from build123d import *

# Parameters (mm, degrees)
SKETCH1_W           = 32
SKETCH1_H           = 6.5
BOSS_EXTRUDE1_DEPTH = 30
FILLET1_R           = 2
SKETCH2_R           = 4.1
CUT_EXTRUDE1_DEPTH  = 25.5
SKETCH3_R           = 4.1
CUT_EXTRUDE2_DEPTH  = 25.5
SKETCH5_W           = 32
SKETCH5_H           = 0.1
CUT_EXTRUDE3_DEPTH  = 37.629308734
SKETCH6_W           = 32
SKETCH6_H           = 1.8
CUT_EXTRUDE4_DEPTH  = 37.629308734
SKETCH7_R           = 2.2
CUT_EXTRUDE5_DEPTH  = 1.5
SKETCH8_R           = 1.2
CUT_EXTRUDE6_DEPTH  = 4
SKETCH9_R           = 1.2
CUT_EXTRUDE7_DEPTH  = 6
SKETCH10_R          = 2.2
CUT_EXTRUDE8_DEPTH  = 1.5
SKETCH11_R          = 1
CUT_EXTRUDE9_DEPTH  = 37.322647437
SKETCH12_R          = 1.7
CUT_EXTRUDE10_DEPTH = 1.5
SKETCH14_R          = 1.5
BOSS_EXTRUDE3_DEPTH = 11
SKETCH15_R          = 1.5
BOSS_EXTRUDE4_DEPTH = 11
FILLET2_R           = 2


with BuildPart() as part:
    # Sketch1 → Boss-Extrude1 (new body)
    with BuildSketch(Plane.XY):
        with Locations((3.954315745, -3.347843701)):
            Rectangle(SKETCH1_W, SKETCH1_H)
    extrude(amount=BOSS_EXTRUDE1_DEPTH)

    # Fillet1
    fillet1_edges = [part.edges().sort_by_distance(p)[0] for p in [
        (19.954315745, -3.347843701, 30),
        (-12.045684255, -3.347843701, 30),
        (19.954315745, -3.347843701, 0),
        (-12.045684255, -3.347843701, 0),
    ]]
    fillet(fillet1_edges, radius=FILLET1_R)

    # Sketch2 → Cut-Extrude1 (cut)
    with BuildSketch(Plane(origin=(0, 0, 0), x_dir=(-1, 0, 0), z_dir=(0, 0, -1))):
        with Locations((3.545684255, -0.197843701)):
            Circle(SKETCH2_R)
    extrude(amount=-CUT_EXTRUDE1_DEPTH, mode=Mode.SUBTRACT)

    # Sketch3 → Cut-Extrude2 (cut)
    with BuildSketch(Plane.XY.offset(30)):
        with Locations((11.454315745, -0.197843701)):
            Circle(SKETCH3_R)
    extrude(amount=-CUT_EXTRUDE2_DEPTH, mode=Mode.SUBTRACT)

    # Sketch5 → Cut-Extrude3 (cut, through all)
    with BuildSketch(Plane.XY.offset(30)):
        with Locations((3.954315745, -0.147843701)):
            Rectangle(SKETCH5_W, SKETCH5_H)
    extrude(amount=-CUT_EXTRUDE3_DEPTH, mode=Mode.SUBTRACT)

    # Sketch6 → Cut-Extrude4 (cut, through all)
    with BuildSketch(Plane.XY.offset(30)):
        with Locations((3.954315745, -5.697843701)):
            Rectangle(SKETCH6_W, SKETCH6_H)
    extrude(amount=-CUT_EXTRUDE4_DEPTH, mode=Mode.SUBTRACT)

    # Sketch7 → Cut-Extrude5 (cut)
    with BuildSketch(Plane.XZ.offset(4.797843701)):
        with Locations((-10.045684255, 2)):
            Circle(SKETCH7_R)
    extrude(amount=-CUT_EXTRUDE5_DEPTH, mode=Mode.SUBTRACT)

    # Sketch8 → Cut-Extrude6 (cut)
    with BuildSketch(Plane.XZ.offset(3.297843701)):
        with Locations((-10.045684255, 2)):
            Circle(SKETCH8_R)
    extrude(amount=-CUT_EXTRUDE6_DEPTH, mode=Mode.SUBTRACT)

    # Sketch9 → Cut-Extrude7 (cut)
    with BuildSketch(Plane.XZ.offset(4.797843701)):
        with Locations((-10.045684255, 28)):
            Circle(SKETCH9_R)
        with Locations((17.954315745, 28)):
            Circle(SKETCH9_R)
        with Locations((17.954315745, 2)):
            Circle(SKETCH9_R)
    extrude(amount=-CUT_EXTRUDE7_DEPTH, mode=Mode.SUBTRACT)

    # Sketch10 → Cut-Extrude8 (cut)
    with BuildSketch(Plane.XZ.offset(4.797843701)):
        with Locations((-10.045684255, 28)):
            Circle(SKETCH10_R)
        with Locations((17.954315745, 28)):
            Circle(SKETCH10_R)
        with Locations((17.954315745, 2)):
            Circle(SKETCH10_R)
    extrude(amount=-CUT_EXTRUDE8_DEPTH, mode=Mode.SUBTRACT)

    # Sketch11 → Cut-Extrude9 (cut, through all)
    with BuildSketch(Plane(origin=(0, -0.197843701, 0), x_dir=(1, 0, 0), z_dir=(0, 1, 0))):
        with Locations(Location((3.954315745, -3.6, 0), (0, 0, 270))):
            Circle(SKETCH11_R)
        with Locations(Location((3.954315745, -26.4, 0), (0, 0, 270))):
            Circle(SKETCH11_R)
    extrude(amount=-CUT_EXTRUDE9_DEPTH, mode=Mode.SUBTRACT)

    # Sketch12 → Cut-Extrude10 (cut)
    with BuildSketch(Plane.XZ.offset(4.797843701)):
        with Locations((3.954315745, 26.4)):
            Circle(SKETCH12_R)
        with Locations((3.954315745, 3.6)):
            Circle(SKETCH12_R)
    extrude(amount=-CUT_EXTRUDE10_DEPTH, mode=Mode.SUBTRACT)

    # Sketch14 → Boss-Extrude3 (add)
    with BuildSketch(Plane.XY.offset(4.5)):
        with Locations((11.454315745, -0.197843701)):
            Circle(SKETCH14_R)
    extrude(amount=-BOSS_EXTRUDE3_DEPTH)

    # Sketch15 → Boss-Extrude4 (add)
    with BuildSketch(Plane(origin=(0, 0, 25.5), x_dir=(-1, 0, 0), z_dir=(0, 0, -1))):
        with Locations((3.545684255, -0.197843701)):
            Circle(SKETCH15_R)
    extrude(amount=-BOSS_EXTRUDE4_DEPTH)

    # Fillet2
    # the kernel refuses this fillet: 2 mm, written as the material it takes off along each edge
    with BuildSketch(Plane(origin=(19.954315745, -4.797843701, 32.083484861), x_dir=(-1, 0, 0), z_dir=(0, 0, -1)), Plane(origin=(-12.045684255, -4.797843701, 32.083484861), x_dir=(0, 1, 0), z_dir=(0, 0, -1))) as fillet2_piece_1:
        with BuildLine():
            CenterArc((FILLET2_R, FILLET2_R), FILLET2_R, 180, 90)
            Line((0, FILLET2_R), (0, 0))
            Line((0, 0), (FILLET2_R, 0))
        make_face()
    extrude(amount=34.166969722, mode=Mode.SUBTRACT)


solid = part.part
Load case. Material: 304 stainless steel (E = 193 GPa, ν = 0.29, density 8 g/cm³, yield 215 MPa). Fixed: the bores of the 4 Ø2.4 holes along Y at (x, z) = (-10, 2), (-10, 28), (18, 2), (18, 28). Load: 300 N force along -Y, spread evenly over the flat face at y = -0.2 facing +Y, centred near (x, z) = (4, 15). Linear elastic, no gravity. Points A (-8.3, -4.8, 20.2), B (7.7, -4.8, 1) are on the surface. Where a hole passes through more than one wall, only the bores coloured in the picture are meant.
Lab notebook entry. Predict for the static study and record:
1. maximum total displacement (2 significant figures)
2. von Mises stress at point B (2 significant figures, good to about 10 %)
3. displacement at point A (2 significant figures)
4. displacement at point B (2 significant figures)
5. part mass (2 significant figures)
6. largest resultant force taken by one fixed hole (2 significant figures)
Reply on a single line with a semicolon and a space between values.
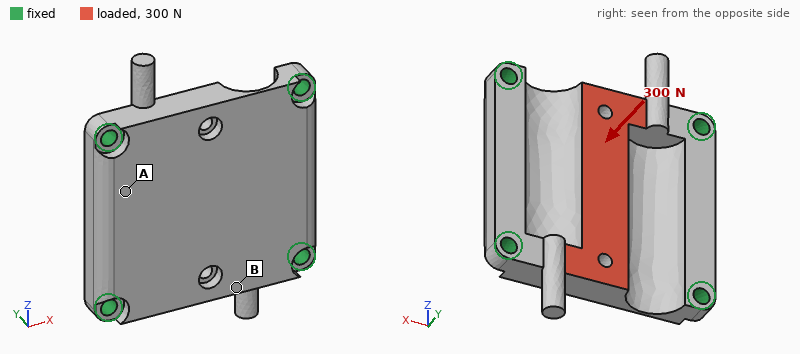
5.7 µm; 14 MPa; 0.88 µm; 3.6 µm; 24 g; 140 N
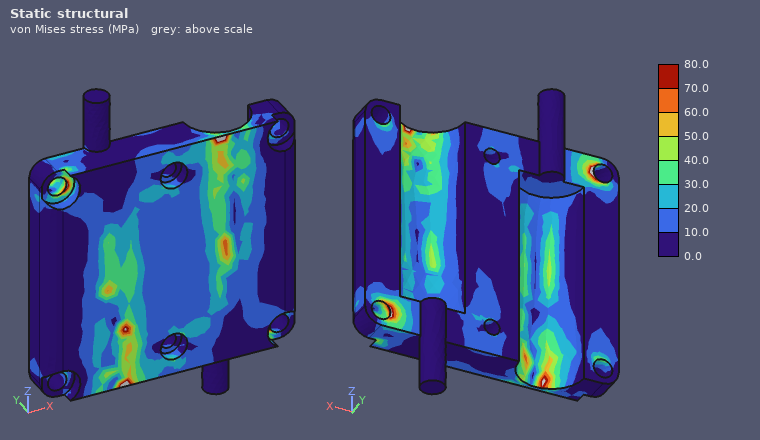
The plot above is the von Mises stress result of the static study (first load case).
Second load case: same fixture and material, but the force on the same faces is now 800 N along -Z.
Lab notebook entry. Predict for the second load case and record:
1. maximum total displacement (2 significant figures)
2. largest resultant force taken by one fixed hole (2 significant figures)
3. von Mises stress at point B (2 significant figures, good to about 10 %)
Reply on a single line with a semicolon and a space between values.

9.3 µm; 240 N; 23 MPa
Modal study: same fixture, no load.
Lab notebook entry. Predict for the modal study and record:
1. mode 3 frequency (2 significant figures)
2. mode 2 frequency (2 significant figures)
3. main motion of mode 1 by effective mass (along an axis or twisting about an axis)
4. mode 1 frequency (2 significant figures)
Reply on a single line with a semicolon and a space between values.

23 kHz; 14 kHz; along Y; 12 kHz
